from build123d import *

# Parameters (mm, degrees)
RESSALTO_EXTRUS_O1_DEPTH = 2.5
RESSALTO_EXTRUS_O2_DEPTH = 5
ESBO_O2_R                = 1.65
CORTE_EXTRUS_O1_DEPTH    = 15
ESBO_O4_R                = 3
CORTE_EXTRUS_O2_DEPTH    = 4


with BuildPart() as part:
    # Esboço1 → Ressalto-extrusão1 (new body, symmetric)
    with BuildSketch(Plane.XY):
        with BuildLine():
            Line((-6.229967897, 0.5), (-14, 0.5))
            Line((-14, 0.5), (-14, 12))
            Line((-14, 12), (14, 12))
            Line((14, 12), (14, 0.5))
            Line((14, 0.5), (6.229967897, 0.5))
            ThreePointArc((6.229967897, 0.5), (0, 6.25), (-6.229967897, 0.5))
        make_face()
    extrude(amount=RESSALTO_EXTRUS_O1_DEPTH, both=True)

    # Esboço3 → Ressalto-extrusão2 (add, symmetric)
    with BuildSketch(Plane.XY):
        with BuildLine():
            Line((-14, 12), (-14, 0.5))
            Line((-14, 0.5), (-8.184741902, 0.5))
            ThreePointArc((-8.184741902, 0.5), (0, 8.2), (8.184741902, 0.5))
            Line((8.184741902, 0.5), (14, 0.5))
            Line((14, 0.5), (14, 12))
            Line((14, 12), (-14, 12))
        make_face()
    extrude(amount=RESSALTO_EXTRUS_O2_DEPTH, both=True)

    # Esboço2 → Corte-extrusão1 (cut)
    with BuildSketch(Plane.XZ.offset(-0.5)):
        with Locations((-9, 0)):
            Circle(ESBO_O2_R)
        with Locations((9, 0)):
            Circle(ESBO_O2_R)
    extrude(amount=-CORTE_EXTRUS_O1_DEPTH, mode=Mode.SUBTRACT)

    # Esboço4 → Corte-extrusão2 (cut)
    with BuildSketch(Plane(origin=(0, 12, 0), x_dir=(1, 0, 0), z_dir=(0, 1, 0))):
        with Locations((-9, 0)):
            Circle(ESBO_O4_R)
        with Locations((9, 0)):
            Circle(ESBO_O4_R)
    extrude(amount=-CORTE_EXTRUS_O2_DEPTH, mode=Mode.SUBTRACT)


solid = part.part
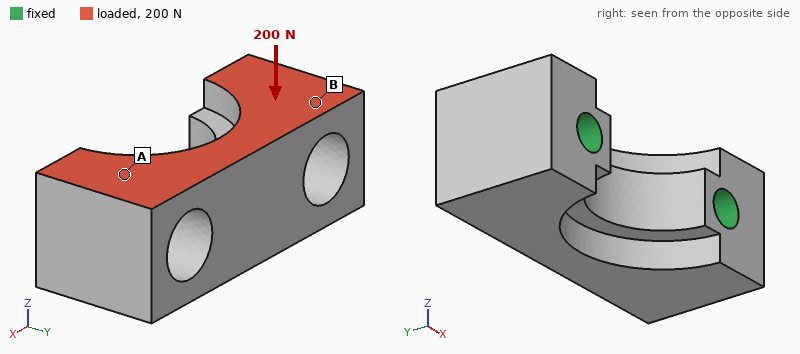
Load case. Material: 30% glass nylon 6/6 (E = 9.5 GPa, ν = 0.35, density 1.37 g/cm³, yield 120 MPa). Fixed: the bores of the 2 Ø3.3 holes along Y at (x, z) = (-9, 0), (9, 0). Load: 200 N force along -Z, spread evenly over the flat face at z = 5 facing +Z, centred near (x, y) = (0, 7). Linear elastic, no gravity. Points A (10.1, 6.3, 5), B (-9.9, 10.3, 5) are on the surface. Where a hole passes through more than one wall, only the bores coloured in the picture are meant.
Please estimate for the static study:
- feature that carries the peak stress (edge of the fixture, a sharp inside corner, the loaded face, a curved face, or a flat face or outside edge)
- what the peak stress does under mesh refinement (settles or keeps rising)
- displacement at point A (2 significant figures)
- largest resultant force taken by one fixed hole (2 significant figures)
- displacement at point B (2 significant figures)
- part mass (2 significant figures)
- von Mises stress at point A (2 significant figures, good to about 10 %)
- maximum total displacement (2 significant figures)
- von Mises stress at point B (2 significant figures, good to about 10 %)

edge of the fixture
keeps rising
1.3 µm
100 N
3.5 µm
2.9 g
2.9 MPa
5.0 µm
0.95 MPa
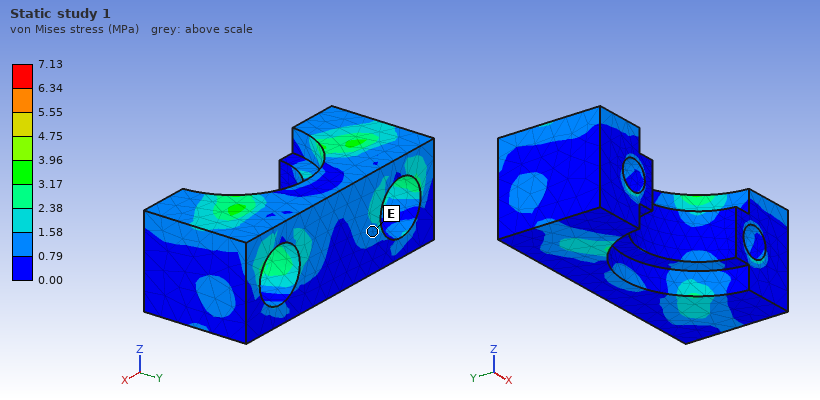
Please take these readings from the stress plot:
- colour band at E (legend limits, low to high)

0.79 to 1.58 MPa
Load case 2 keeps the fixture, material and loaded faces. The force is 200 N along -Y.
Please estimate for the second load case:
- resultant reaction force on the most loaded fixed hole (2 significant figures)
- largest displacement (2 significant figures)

100 N
8.1 µm
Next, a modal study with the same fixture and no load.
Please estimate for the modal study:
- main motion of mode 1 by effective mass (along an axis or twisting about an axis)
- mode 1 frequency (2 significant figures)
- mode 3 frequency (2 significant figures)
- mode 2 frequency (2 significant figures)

along Z
23 kHz
35 kHz
34 kHz
